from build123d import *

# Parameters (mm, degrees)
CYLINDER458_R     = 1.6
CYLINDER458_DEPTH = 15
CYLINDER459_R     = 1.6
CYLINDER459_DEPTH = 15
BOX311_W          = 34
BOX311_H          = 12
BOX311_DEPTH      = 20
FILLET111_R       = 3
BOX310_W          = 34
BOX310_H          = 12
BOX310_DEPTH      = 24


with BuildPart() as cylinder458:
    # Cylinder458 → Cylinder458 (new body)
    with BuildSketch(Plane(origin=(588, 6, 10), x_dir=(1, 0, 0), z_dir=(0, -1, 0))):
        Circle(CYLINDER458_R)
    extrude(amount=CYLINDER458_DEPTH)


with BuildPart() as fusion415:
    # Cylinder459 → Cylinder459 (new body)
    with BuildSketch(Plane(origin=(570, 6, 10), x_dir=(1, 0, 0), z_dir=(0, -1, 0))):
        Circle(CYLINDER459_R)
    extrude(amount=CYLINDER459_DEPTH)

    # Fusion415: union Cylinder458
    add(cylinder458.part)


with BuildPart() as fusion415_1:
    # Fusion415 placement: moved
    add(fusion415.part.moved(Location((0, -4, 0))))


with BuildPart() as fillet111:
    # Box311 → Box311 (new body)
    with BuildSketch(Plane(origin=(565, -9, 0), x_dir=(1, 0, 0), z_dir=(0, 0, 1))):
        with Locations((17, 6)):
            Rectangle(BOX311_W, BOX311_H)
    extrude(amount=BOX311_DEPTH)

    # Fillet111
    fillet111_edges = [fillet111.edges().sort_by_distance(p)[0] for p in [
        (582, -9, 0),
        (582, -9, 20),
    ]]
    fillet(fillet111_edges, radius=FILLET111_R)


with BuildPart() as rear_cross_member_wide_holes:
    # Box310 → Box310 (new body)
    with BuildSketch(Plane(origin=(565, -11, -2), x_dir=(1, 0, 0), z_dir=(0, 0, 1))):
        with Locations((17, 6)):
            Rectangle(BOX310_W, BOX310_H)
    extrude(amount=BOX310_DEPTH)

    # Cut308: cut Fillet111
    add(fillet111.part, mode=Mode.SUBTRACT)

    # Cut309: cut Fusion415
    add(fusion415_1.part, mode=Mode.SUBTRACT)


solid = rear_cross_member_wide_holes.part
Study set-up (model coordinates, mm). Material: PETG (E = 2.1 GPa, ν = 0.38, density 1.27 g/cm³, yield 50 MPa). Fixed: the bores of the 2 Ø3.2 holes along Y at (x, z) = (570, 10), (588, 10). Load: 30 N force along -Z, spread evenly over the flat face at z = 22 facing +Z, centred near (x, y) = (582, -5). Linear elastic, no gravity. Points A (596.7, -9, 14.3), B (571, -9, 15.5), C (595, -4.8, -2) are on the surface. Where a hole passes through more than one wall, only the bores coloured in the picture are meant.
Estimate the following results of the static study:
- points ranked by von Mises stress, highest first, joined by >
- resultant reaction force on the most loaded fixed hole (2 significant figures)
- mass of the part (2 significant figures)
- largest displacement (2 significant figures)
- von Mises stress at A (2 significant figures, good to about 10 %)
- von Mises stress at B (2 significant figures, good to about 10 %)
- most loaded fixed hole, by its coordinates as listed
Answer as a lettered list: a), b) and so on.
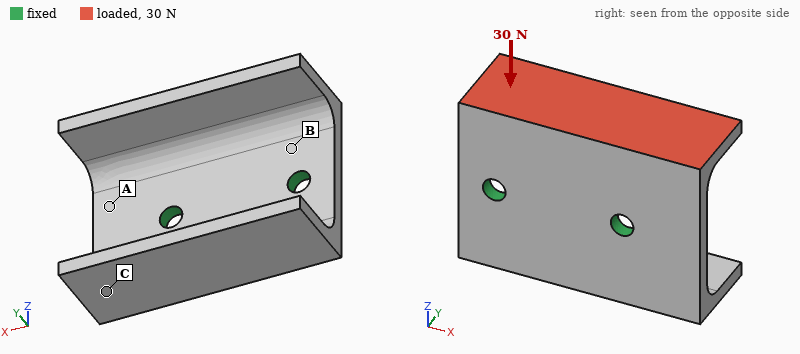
a) B > A > C
b) 20 N
c) 3.9 g
d) 0.39 mm
e) 5.2 MPa
f) 6.7 MPa
g) (588, 10)
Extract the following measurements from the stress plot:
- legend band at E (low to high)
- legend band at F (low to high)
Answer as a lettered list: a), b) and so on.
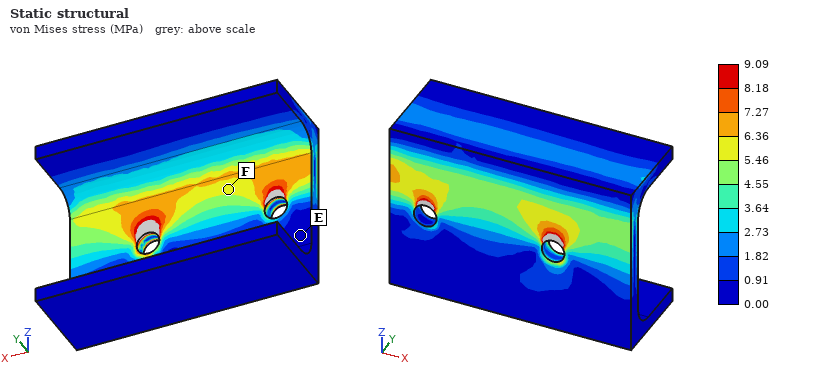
a) 0.00 to 0.91 MPa
b) 5.46 to 6.36 MPa
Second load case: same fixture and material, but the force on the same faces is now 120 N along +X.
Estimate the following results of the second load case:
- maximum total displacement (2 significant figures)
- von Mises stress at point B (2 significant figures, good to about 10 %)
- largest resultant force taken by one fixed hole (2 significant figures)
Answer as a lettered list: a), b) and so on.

a) 0.49 mm
b) 10 MPa
c) 100 N
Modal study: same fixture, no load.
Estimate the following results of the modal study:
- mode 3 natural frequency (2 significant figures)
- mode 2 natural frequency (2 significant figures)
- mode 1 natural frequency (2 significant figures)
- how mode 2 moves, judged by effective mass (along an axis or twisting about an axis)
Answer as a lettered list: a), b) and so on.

a) 1800 Hz
b) 1300 Hz
c) 1100 Hz
d) along Y
